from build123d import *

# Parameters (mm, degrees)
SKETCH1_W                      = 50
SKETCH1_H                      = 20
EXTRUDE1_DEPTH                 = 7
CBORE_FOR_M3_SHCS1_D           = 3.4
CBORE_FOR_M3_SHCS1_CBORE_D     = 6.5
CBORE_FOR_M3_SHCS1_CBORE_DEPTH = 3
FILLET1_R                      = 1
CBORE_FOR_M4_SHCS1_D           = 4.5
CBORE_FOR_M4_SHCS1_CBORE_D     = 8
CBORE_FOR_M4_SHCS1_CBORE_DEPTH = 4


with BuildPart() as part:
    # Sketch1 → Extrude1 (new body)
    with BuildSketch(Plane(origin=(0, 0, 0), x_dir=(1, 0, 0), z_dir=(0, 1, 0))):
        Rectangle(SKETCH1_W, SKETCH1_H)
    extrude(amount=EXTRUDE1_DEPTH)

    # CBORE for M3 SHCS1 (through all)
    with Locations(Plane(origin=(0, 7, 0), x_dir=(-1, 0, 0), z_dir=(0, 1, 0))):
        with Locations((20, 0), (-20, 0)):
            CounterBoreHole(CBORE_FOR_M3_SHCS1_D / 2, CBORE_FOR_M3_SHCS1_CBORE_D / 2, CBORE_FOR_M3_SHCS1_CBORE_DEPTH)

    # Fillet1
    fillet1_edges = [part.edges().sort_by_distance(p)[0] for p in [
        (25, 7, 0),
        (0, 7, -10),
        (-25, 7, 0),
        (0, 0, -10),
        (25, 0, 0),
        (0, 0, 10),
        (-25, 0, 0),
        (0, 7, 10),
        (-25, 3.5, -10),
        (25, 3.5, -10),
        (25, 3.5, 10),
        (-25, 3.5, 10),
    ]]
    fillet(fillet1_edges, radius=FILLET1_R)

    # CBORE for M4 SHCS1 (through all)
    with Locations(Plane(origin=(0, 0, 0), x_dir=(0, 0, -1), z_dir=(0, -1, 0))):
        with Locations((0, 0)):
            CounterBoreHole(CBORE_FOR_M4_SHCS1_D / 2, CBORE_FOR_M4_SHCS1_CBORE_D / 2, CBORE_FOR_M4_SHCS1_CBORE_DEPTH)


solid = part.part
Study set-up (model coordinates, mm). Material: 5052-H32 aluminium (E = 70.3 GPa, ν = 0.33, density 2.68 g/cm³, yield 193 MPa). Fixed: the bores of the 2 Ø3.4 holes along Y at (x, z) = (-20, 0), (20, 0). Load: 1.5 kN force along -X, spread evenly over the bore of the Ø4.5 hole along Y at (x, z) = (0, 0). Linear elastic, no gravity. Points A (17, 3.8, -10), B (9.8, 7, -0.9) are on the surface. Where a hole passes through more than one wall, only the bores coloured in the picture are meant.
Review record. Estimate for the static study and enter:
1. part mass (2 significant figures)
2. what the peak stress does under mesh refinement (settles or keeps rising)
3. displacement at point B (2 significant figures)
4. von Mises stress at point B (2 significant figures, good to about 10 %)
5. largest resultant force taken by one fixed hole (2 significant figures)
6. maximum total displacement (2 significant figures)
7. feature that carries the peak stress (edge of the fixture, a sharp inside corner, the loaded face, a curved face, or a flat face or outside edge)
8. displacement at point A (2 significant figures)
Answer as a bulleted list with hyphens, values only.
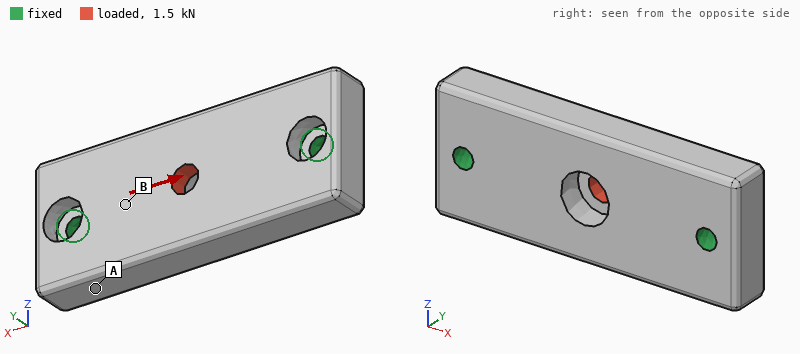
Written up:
- 17 g
- keeps rising
- 2.1 µm
- 13 MPa
- 760 N
- 4.6 µm
- a sharp inside corner
- 1.6 µm
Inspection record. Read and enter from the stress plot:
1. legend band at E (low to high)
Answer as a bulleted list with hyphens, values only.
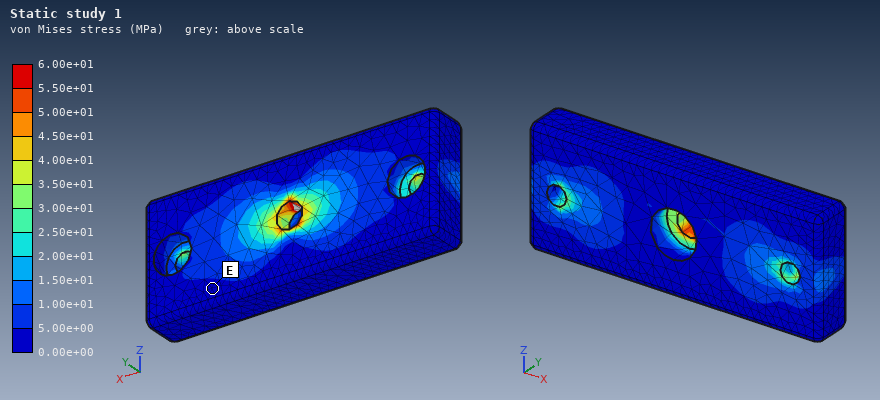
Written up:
- 0.00e+00 to 5.00e+00 MPa
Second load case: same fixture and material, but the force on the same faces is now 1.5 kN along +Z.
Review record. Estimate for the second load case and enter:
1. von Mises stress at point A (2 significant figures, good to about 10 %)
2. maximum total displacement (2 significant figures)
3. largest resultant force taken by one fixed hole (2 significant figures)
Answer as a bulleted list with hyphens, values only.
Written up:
- 7.2 MPa
- 20 µm
- 750 N
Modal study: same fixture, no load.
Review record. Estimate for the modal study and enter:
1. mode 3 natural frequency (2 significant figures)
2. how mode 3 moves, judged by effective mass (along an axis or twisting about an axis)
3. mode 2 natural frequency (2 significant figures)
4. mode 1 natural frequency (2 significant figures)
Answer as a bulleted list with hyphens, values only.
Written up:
- 24 kHz
- along Z
- 14 kHz
- 14 kHz
